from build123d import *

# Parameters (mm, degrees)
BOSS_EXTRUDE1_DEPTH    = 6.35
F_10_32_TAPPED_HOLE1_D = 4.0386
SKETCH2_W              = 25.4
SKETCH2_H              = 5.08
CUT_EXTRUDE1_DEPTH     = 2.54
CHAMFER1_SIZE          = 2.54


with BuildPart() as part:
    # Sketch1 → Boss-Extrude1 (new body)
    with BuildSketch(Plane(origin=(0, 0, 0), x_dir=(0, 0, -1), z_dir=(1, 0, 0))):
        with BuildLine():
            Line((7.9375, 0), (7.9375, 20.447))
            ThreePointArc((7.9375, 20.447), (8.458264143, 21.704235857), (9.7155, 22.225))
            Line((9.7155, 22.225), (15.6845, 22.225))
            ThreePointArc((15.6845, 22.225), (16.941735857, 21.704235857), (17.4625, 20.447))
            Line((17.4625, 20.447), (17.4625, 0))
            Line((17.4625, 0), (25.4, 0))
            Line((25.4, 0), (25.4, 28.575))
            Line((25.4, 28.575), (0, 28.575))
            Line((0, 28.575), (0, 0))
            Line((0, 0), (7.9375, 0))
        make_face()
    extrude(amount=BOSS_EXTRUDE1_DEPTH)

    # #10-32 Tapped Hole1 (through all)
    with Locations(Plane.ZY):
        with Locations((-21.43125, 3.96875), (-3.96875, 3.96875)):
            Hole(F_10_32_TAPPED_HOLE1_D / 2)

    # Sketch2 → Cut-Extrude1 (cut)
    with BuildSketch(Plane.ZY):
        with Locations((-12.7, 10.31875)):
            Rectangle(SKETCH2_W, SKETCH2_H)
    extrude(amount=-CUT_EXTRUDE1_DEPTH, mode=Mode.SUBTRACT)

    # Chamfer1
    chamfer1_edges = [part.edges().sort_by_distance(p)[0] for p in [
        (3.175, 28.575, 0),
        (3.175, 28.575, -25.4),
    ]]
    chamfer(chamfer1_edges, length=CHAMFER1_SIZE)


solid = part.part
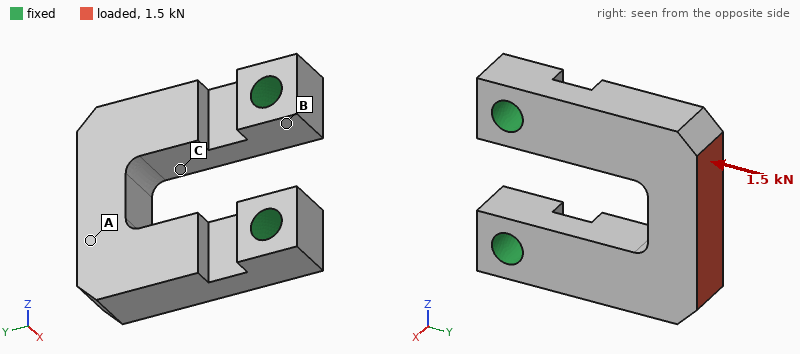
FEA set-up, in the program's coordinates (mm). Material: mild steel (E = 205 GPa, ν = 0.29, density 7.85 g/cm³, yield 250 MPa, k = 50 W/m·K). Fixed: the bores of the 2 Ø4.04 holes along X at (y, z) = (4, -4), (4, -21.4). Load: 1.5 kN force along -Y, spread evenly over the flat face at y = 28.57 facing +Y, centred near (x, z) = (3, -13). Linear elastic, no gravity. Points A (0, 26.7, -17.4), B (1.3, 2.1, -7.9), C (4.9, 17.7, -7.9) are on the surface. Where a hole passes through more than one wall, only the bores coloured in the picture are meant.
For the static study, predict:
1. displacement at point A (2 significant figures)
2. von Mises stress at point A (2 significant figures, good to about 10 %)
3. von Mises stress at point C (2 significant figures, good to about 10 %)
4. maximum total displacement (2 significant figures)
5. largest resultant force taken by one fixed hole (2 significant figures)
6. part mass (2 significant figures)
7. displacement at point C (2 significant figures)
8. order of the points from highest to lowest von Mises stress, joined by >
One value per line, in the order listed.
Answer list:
17 µm
16 MPa
30 MPa
19 µm
760 N
22 g
7.2 µm
C > A > B
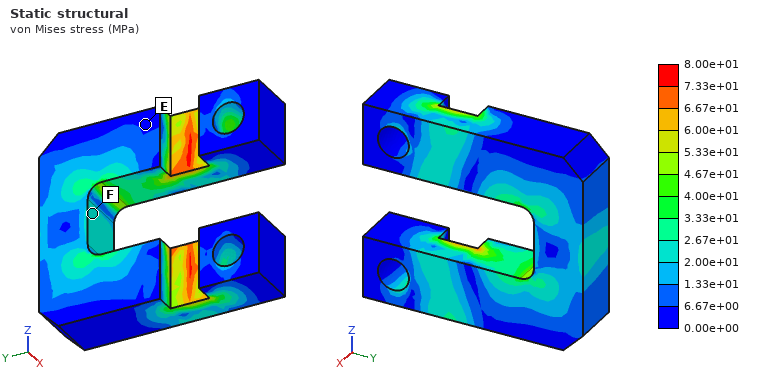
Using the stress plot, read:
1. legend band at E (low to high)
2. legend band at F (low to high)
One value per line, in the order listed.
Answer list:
0.00e+00 to 6.67e+00 MPa
2.00e+01 to 2.67e+01 MPa
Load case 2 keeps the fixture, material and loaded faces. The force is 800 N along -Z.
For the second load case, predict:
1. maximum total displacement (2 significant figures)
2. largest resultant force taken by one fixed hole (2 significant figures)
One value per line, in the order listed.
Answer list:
15 µm
750 N
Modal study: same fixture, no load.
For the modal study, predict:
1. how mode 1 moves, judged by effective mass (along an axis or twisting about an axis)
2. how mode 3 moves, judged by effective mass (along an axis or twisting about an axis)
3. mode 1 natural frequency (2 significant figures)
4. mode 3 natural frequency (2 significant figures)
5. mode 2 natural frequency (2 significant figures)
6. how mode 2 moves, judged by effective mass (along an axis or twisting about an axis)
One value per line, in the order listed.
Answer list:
along X
along Z
4300 Hz
12 kHz
11 kHz
along Z
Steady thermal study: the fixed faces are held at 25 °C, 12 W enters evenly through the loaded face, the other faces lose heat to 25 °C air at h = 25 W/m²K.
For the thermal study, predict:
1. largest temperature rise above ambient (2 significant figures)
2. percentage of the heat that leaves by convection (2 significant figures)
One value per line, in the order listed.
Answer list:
64 K
11 %
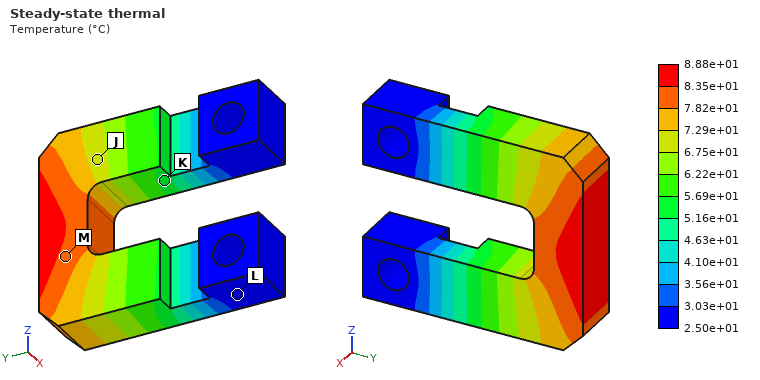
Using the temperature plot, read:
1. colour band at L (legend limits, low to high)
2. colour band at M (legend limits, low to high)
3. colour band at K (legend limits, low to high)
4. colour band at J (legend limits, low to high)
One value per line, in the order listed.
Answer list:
2.50e+01 to 3.03e+01 °C
7.82e+01 to 8.35e+01 °C
5.16e+01 to 5.69e+01 °C
6.75e+01 to 7.29e+01 °C
